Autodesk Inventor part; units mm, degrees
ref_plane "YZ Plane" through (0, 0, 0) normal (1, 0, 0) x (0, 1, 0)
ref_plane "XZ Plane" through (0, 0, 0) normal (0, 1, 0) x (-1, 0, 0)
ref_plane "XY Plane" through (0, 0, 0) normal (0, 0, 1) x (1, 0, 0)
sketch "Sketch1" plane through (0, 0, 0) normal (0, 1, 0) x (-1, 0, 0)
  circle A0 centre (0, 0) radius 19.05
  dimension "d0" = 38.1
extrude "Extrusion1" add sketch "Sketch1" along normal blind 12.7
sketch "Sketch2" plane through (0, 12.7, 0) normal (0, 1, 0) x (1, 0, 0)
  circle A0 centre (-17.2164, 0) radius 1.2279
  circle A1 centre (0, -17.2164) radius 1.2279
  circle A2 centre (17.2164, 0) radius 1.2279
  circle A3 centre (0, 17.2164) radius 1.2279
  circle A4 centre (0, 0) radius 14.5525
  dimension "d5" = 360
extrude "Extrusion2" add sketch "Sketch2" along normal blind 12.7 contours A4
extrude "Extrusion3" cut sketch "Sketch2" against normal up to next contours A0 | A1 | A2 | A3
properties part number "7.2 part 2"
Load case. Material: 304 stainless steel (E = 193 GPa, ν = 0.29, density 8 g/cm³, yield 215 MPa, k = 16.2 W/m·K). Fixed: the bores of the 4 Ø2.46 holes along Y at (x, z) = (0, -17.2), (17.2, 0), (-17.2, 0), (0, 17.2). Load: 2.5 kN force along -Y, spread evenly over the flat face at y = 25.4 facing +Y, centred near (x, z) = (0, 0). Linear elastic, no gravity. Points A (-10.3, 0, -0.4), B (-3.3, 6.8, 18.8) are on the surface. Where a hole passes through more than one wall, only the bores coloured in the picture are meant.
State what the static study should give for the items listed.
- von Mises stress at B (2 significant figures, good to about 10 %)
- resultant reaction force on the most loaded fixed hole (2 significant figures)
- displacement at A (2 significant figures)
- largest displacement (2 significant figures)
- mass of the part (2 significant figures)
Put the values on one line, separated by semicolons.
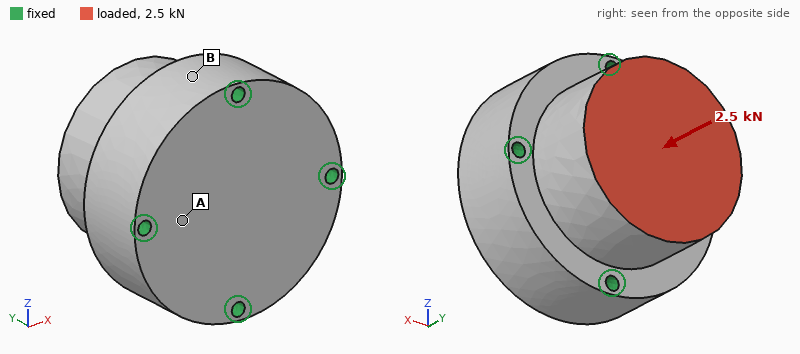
4.9 MPa; 640 N; 0.36 µm; 0.70 µm; 180 g
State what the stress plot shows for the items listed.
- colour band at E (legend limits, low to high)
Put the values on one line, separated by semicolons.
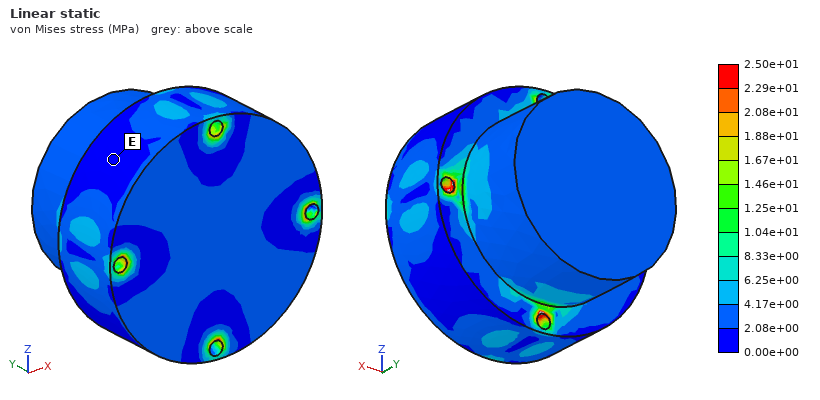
0.00e+00 to 2.08e+00 MPa
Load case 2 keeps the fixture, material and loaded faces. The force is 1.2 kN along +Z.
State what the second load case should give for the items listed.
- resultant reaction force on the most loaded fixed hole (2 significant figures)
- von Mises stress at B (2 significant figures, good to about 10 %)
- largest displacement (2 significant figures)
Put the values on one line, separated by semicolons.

710 N; 6.3 MPa; 1.3 µm
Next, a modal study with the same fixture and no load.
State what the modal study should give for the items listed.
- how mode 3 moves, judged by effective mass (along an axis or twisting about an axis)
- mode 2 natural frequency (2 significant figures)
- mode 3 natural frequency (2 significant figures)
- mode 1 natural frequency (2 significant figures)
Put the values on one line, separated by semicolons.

along Y; 26 kHz; 30 kHz; 26 kHz
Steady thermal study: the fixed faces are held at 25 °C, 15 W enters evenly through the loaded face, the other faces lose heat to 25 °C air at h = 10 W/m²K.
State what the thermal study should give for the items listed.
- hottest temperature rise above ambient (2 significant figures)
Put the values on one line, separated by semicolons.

31 K
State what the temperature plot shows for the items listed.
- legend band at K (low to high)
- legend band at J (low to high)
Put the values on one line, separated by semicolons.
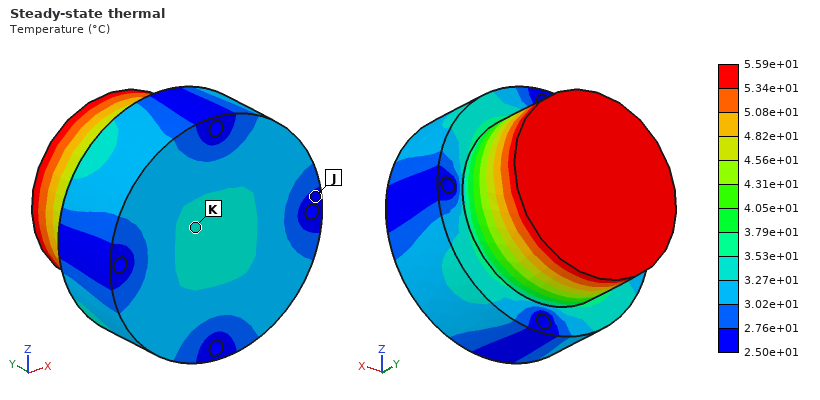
3.27e+01 to 3.53e+01 °C; 2.50e+01 to 2.76e+01 °C
